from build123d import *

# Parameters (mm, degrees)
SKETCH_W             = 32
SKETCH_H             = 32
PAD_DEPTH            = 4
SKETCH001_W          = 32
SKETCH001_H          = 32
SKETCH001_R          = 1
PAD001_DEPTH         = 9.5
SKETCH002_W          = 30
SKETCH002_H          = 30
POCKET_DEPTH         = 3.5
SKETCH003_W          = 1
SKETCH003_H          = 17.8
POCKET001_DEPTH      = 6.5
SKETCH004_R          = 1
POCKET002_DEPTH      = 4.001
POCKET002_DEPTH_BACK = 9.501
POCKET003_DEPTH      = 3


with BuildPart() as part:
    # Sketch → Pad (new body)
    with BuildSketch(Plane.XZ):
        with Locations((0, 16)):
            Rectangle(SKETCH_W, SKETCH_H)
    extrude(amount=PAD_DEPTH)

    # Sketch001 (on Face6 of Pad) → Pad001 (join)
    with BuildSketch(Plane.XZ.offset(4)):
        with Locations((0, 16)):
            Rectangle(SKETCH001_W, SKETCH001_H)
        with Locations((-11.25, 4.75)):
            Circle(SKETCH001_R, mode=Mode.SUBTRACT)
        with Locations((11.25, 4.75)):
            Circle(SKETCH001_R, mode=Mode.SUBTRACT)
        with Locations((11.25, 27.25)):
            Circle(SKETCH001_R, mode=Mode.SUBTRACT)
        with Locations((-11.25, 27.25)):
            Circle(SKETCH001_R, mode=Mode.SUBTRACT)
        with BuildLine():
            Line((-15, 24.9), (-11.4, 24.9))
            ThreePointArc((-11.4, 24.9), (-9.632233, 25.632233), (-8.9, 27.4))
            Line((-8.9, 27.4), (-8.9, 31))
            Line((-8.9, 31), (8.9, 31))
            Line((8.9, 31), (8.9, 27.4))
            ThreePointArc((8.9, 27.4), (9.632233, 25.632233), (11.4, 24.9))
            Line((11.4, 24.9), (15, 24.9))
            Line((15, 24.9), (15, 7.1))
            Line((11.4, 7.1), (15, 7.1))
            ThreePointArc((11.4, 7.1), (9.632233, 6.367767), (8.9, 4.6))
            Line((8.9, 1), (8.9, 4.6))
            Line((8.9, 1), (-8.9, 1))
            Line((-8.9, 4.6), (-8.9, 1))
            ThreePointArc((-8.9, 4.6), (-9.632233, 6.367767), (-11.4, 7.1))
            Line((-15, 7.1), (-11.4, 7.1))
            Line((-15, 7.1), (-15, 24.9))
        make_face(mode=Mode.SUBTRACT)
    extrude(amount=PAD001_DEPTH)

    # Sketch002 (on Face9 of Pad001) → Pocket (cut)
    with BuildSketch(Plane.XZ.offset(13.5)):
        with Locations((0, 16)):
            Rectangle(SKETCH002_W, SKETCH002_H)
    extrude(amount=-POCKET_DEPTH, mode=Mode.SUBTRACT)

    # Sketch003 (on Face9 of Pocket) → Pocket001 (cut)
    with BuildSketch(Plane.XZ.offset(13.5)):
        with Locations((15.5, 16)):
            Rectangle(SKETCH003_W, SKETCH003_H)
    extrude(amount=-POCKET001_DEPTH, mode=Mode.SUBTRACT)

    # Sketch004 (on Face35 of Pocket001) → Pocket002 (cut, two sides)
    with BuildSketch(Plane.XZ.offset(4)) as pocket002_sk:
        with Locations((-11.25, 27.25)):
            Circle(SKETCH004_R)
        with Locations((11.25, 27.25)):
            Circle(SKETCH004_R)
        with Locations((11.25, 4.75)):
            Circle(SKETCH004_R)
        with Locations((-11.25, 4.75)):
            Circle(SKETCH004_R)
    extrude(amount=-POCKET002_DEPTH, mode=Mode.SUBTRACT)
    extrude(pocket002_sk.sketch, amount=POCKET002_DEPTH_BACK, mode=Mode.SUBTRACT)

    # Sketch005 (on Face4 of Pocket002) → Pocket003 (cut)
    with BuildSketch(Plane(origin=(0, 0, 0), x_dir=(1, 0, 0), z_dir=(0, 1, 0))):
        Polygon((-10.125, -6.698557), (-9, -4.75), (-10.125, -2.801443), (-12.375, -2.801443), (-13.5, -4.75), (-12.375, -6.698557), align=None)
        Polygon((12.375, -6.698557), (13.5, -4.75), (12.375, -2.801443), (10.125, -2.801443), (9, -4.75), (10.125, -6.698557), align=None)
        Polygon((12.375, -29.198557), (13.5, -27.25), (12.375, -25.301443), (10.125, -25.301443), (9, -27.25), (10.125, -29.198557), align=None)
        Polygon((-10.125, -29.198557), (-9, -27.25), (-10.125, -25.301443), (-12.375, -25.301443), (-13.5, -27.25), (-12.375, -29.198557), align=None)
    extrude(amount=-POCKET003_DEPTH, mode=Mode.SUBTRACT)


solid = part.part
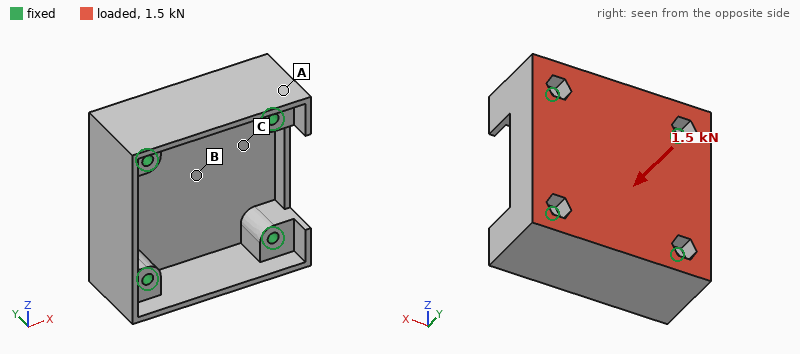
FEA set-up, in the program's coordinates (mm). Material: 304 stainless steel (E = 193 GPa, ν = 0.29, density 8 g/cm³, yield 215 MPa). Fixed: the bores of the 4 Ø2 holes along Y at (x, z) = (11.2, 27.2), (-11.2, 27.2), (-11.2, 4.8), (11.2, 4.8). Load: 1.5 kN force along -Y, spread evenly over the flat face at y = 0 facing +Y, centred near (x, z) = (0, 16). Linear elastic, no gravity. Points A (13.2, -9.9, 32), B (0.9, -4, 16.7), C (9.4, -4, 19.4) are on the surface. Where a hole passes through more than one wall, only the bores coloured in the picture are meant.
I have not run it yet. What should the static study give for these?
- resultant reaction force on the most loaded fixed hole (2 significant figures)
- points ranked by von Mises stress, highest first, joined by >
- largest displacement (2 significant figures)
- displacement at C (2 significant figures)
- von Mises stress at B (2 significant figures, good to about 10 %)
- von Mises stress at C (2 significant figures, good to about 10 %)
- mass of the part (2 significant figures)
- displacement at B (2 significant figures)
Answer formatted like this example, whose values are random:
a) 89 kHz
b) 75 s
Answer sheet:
a) 430 N
b) B > C > A
c) 3.3 µm
d) 2.0 µm
e) 15 MPa
f) 8.3 MPa
g) 46 g
h) 3.3 µm
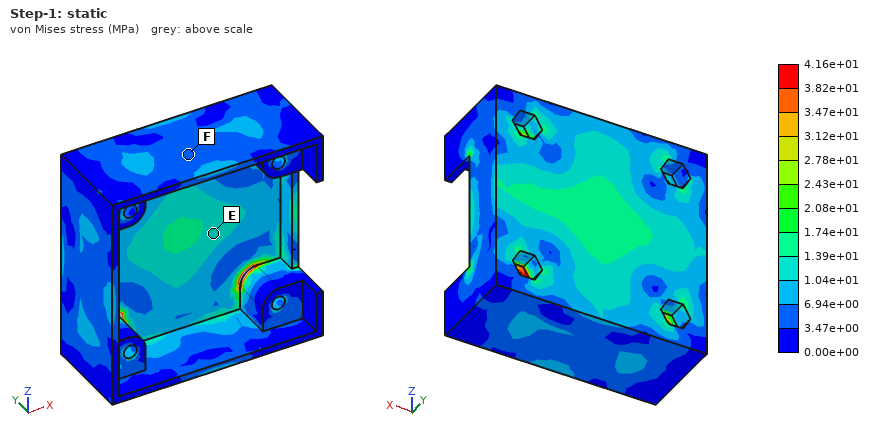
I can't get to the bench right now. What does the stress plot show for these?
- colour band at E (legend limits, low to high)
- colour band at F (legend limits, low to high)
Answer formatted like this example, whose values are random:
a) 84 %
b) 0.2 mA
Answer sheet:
a) 1.04e+01 to 1.39e+01 MPa
b) 3.47e+00 to 6.94e+00 MPa
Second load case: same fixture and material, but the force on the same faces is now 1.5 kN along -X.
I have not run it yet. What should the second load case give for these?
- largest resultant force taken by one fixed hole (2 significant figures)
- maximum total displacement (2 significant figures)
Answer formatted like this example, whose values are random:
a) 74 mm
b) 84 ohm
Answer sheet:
a) 400 N
b) 1.2 µm
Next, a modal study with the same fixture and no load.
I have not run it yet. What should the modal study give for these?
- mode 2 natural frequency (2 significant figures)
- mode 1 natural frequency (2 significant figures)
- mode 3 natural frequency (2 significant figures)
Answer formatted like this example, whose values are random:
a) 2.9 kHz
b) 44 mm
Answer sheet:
a) 16 kHz
b) 16 kHz
c) 16 kHz
